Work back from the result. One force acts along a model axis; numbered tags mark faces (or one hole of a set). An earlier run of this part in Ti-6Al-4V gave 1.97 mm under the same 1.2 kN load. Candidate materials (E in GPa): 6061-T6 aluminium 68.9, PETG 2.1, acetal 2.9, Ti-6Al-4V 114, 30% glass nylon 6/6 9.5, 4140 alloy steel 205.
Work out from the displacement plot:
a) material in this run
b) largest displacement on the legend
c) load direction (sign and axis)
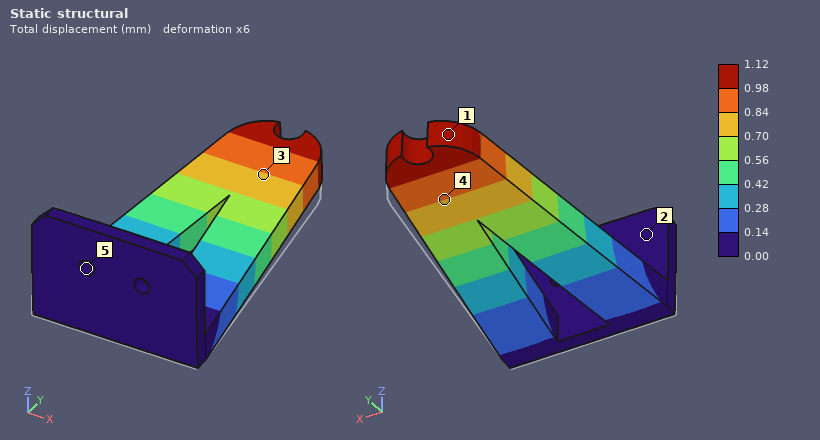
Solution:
4140 alloy steel
1.12 mm
+Z
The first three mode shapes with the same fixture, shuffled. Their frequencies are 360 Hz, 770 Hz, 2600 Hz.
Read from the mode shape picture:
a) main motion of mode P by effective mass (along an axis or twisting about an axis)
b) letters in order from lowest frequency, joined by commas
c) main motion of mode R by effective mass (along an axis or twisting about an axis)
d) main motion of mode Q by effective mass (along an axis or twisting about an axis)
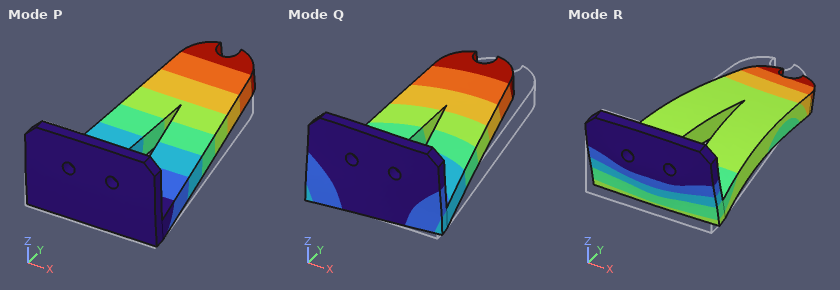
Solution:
along Z
P, Q, R
along Y
along X
